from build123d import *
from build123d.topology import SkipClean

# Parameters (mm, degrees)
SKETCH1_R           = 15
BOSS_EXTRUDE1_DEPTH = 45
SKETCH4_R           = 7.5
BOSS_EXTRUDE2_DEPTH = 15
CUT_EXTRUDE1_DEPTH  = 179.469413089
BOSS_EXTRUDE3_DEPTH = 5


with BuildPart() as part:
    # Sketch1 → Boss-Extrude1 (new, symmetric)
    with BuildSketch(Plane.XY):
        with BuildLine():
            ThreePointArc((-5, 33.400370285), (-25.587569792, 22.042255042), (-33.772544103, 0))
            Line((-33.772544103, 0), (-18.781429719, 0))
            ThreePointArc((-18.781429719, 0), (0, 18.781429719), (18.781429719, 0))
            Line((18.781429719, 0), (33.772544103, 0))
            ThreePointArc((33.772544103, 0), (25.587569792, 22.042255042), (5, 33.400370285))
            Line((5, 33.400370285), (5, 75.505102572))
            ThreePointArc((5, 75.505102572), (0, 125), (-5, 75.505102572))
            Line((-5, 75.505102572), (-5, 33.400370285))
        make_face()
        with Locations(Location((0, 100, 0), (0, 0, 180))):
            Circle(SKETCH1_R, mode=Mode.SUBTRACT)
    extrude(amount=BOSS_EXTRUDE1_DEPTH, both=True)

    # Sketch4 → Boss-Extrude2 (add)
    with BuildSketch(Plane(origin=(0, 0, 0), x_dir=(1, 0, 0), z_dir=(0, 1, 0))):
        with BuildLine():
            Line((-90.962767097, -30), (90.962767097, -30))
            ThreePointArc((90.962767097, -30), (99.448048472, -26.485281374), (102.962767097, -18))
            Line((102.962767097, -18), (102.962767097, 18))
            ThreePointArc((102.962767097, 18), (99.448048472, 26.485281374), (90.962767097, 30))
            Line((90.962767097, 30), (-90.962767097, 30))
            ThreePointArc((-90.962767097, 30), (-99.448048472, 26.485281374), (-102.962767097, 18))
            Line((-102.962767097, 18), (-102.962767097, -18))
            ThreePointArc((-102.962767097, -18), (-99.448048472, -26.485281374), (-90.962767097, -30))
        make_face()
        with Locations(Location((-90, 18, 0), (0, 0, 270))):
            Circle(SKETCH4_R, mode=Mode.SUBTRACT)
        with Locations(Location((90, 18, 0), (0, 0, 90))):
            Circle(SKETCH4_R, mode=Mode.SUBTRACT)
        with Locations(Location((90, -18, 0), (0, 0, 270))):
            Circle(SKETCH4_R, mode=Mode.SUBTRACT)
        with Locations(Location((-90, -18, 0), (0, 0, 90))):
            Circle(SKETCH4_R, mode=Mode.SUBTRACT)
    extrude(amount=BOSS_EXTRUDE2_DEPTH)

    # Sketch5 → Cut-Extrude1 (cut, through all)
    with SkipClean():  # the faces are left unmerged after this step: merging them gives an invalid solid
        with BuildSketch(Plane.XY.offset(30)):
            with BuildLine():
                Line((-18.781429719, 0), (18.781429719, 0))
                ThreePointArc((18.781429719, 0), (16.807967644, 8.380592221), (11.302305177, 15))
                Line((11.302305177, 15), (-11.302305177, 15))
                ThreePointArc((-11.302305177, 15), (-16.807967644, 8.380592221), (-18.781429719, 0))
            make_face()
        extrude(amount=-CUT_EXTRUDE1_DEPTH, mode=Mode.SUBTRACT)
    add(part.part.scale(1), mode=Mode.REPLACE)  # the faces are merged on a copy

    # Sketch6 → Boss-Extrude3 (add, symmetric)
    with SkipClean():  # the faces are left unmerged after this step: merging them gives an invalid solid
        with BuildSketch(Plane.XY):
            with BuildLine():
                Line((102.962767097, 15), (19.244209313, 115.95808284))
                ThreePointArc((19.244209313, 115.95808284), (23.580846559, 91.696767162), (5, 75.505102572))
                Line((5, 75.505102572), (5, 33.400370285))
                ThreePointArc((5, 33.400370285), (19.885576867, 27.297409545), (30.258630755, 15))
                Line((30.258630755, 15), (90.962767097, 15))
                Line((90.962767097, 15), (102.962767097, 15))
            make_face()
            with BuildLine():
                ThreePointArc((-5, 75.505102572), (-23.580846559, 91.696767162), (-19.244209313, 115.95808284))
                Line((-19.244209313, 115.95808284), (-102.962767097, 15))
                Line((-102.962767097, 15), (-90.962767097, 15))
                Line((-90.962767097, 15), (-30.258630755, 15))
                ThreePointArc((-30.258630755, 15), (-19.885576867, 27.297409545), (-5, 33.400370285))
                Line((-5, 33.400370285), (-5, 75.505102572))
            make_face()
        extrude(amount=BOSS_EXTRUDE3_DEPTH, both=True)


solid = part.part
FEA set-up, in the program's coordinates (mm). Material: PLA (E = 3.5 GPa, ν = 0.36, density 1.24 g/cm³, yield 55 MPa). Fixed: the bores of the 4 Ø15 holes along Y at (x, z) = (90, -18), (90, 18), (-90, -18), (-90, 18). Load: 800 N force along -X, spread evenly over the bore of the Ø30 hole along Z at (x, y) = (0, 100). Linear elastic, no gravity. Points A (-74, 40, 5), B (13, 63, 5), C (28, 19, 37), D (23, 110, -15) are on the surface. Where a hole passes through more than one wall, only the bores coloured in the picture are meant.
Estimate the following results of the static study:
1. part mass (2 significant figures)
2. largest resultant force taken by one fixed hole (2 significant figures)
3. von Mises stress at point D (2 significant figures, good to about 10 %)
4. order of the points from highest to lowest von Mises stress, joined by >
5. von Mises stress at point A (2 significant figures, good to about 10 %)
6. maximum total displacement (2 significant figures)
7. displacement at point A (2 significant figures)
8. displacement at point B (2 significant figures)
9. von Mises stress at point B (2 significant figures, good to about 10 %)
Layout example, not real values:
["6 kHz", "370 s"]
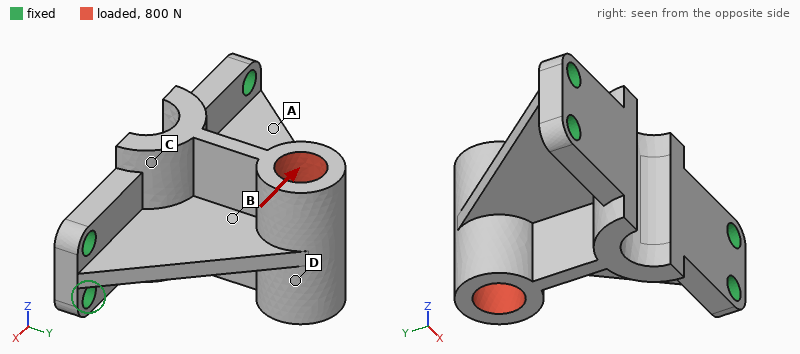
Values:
["580 g", "310 N", "0.42 MPa", "A > B > D > C", "1.6 MPa", "97 µm", "18 µm", "31 µm", "0.86 MPa"]
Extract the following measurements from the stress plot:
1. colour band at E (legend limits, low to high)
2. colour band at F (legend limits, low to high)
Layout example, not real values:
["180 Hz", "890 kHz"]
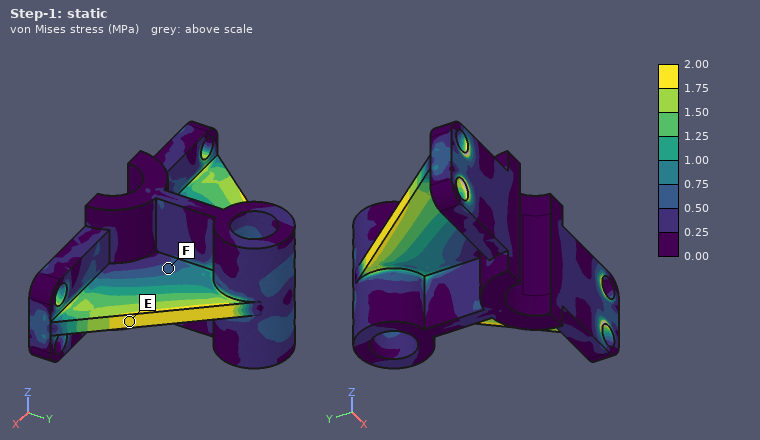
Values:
["1.75 to 2.00 MPa", "0.50 to 0.75 MPa"]
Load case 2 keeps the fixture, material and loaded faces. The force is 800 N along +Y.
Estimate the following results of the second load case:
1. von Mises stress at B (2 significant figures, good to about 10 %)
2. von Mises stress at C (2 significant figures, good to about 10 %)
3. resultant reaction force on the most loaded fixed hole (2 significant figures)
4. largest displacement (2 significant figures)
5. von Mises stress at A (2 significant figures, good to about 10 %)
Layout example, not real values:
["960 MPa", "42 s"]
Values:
["0.57 MPa", "0.22 MPa", "300 N", "55 µm", "1.1 MPa"]
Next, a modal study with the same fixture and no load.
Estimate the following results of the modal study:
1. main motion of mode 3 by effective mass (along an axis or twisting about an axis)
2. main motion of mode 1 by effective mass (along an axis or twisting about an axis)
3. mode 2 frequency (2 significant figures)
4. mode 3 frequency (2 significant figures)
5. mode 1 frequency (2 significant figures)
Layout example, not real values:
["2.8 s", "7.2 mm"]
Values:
["along Y", "along Z", "750 Hz", "1000 Hz", "240 Hz"]
